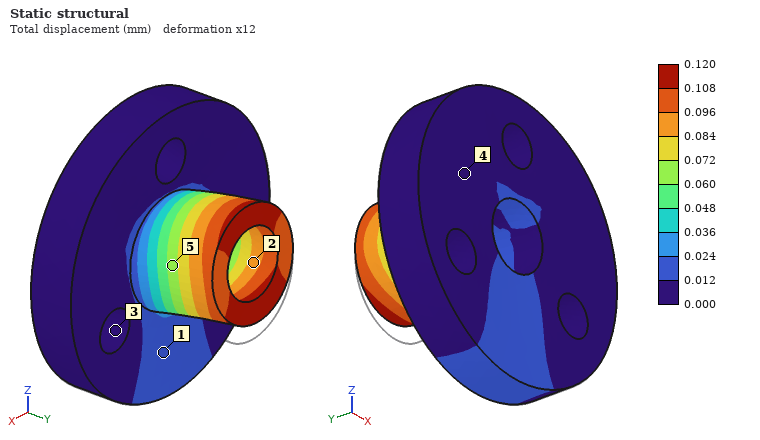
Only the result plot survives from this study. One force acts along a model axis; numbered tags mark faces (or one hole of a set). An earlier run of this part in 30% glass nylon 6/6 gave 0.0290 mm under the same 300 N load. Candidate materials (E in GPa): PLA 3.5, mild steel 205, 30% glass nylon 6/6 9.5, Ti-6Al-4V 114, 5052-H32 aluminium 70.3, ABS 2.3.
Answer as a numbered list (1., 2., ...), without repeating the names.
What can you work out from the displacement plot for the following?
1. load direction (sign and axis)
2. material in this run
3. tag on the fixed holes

1. +Z
2. ABS
3. 3
